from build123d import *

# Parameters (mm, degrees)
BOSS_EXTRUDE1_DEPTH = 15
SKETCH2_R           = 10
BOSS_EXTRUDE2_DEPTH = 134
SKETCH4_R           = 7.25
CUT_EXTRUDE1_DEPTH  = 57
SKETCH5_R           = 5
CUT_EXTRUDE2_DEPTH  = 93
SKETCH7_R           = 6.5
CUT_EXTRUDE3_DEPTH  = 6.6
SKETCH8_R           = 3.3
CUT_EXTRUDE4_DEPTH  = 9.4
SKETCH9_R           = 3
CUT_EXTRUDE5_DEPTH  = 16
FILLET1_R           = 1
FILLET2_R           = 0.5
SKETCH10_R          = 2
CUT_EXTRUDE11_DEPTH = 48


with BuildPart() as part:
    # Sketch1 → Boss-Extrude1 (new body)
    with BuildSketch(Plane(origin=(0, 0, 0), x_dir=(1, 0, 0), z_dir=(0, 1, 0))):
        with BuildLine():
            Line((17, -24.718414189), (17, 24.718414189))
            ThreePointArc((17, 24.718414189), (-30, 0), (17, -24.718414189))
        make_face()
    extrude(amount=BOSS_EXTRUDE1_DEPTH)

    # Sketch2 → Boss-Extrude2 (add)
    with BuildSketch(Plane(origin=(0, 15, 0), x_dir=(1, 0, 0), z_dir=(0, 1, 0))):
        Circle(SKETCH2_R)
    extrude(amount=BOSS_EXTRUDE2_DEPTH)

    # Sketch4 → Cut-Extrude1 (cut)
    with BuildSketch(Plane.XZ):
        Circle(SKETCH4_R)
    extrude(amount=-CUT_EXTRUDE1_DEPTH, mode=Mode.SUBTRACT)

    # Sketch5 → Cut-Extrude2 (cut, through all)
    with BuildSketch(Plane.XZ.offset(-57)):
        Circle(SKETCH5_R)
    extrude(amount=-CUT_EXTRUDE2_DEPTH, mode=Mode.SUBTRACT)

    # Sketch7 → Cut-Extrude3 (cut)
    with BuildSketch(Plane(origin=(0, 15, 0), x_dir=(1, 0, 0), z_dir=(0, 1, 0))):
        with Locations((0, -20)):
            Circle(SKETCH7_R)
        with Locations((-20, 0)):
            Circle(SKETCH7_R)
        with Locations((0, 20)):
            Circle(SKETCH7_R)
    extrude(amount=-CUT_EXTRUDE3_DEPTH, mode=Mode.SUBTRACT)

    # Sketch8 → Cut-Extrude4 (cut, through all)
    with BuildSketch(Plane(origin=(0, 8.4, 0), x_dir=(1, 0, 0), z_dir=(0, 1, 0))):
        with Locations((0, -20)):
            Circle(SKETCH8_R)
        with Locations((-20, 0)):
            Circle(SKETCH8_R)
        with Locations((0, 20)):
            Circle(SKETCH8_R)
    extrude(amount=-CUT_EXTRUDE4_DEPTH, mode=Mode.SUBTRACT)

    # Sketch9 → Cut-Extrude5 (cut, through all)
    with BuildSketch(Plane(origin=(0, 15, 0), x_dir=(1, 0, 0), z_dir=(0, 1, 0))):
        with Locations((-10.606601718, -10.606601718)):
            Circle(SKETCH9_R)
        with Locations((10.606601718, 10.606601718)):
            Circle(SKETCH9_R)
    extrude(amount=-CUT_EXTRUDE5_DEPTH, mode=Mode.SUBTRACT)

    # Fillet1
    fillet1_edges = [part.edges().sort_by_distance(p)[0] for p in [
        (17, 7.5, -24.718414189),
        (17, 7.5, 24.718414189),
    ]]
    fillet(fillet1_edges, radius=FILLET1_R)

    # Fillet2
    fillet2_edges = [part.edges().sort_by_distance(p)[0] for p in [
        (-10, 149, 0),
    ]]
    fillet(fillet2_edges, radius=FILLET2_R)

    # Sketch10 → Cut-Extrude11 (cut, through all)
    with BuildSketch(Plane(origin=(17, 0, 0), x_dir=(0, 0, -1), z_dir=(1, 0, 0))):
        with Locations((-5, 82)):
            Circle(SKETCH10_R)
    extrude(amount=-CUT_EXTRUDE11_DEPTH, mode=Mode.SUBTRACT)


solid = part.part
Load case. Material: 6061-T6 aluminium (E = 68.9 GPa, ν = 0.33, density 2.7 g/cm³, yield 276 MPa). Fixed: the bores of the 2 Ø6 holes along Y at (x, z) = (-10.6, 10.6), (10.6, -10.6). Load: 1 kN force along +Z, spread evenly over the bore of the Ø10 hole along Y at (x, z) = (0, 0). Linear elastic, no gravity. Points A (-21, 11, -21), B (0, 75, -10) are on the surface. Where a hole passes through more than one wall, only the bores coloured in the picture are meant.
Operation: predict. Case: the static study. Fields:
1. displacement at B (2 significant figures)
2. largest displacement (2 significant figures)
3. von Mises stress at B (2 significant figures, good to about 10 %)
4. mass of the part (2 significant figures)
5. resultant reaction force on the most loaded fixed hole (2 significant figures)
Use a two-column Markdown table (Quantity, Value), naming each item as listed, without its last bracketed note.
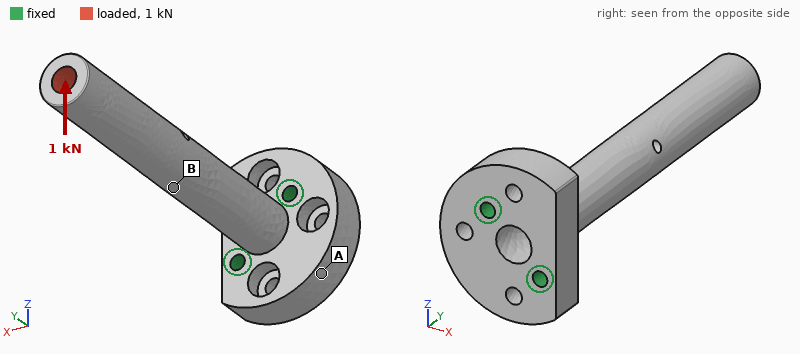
| Quantity | Value |
|---|---|
| displacement at B | 0.44 mm |
| largest displacement | 1.3 mm |
| von Mises stress at B | 42 MPa |
| mass of the part | 150 g |
| resultant reaction force on the most loaded fixed hole | 2.8 kN |
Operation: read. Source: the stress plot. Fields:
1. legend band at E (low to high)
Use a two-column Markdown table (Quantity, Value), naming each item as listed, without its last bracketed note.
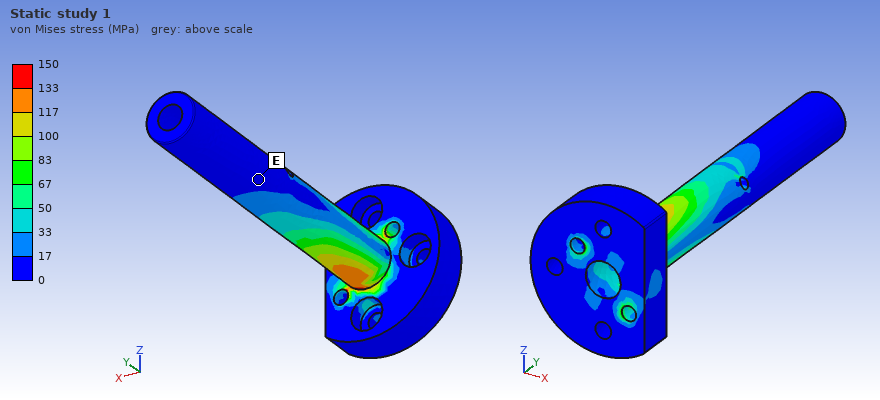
| Quantity | Value |
|---|---|
| legend band at E | 0 to 17 MPa |
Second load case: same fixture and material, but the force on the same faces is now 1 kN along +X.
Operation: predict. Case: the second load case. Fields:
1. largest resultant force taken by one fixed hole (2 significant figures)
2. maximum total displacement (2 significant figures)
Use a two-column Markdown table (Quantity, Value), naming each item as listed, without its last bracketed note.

| Quantity | Value |
|---|---|
| largest resultant force taken by one fixed hole | 2.9 kN |
| maximum total displacement | 1.3 mm |
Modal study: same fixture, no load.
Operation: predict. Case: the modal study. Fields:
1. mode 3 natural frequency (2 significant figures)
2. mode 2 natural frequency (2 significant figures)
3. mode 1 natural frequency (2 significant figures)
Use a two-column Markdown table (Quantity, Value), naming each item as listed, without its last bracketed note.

| Quantity | Value |
|---|---|
| mode 3 natural frequency | 4200 Hz |
| mode 2 natural frequency | 730 Hz |
| mode 1 natural frequency | 690 Hz |
